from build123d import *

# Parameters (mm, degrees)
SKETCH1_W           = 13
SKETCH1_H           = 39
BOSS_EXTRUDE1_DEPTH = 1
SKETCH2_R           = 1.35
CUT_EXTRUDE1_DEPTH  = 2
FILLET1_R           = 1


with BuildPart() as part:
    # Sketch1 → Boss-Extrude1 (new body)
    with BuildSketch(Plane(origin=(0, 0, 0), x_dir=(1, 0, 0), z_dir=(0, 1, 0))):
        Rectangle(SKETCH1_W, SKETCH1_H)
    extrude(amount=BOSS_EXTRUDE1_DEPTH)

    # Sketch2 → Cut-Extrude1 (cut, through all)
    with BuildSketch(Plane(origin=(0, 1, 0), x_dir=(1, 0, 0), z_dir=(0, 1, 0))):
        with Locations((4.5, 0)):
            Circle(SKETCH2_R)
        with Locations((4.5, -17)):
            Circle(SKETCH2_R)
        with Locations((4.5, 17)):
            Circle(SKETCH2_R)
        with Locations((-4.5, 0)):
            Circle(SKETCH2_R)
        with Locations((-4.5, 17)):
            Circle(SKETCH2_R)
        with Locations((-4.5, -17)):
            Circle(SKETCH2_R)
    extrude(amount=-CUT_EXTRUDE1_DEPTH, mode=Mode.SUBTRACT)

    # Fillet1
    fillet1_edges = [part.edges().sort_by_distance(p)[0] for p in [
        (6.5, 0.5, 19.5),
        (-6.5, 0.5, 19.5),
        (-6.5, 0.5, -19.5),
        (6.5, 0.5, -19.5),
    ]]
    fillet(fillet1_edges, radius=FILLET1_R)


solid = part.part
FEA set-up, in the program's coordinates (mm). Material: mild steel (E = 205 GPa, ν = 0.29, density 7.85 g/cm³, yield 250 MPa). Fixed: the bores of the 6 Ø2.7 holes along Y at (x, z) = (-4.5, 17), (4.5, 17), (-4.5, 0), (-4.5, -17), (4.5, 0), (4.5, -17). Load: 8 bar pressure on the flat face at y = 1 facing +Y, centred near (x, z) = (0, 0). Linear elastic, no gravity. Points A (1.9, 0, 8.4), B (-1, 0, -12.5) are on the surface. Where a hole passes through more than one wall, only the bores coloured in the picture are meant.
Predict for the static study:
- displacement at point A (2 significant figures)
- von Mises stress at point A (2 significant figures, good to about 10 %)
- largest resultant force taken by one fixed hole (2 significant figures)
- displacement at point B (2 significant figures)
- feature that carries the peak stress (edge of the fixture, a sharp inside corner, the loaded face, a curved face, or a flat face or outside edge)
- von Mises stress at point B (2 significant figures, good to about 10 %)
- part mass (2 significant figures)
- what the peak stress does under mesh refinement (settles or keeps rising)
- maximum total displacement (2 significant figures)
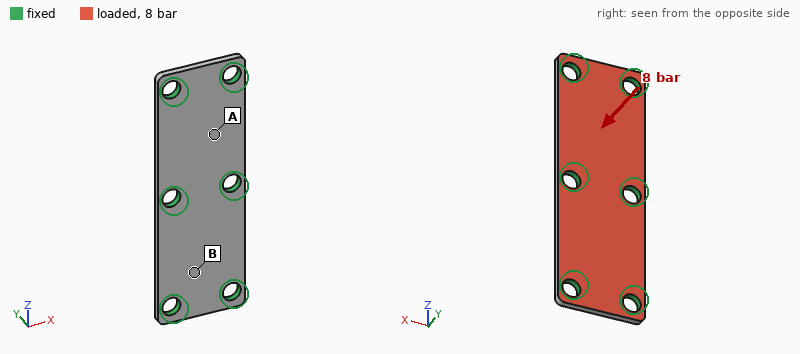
6.9 µm
41 MPa
84 N
4.3 µm
edge of the fixture
14 MPa
3.7 g
keeps rising
7.0 µm
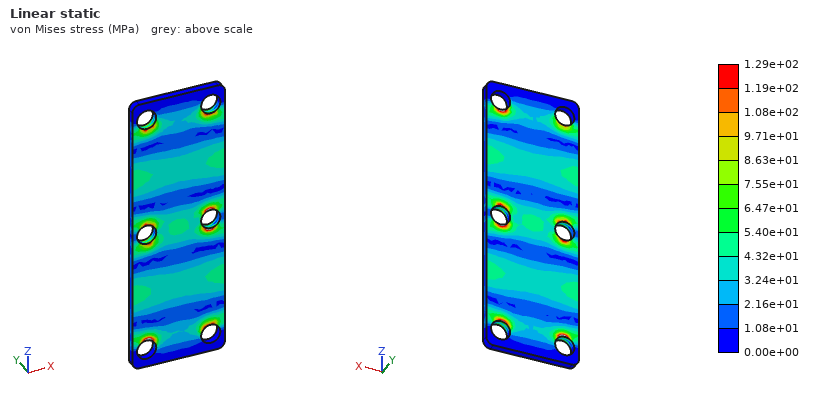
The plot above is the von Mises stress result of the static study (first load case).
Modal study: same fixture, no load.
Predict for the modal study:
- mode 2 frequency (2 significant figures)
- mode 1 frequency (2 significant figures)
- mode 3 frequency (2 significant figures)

22 kHz
22 kHz
29 kHz
